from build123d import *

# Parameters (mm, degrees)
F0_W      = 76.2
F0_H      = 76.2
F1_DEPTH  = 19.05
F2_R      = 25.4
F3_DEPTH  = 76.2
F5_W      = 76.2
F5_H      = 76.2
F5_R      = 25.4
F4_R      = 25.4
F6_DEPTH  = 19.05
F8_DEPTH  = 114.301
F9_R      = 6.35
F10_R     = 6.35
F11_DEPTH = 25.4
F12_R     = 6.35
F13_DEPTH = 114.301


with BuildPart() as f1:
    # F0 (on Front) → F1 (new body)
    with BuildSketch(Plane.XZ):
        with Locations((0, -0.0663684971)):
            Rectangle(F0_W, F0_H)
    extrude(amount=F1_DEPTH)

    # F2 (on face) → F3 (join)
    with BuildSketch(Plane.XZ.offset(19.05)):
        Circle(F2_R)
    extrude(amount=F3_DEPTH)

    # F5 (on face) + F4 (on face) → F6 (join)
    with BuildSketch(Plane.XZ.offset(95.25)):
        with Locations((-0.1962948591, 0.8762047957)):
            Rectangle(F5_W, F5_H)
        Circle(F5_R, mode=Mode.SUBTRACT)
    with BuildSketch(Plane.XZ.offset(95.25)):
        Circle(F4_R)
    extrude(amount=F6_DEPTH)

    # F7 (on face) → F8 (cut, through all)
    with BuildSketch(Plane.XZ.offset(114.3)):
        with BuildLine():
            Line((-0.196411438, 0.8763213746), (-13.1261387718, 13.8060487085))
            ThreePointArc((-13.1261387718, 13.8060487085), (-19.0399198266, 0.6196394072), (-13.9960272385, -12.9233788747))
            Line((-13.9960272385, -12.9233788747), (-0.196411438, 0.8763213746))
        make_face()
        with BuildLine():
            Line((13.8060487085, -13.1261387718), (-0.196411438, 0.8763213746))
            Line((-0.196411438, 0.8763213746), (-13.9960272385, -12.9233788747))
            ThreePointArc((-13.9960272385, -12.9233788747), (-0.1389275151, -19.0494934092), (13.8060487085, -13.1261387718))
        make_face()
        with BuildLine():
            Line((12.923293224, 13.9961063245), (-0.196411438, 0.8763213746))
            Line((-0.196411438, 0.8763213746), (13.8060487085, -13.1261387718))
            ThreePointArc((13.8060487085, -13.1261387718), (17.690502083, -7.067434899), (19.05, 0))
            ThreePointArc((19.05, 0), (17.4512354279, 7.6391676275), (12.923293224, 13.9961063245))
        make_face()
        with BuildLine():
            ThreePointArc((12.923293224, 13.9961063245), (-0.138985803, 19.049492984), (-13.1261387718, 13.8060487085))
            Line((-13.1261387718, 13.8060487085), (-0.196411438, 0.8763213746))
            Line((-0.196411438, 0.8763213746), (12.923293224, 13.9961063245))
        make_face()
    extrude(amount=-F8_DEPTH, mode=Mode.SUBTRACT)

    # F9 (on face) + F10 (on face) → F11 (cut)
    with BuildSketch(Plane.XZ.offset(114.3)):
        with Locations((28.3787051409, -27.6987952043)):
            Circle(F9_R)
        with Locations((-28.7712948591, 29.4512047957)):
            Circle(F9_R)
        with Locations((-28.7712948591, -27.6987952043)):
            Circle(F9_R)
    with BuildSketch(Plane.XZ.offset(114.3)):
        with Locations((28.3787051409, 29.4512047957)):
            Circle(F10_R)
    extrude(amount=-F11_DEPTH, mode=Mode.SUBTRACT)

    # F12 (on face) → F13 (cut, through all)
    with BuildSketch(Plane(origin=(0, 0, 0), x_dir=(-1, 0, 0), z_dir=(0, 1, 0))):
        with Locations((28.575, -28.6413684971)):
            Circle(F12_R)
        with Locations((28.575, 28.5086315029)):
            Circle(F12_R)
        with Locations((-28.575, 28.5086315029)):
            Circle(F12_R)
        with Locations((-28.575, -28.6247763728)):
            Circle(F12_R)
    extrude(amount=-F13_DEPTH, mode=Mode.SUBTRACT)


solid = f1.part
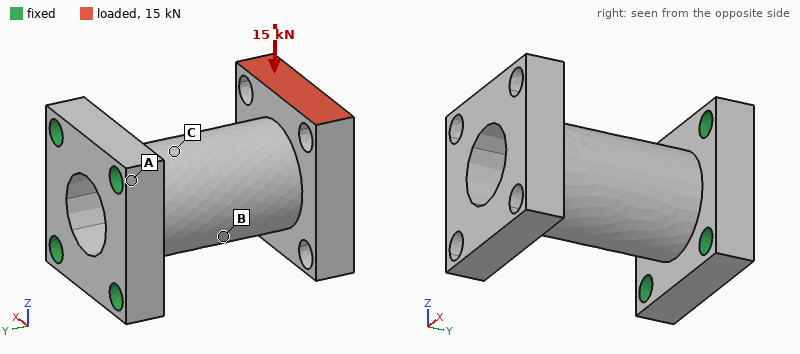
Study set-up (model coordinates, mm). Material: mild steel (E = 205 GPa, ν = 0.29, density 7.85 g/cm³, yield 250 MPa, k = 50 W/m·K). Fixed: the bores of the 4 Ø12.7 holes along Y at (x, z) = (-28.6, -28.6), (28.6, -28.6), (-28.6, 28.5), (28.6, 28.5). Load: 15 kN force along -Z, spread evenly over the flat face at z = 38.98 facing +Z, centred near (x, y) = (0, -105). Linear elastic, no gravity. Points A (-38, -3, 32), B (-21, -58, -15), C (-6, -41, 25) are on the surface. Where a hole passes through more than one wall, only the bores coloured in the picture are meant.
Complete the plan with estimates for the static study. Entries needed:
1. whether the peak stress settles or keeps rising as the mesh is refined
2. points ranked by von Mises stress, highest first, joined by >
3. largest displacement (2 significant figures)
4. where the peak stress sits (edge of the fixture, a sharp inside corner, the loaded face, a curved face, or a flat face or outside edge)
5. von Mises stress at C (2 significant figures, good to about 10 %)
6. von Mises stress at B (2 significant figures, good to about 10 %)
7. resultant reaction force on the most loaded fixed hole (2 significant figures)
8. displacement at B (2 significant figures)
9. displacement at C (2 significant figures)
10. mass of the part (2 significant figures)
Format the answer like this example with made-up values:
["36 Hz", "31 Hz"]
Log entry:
["keeps rising", "C > B > A", "0.18 mm", "edge of the fixture", "99 MPa", "65 MPa", "15 kN", "0.058 mm", "0.040 mm", "1.8 kg"]
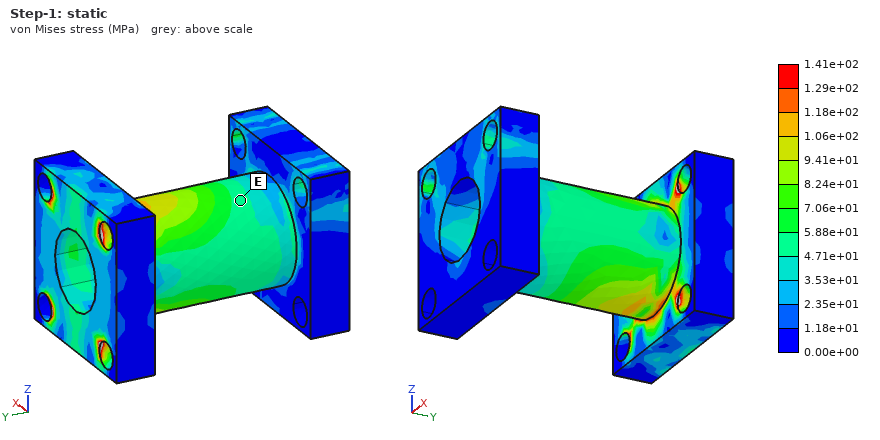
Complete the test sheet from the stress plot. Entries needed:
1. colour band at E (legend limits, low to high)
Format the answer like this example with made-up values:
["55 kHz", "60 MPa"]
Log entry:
["4.71e+01 to 5.88e+01 MPa"]
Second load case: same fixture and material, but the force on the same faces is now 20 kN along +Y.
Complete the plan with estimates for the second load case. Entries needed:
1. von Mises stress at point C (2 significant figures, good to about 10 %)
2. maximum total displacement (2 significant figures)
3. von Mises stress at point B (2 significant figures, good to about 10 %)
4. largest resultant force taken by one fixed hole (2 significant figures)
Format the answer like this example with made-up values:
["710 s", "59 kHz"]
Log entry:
["100 MPa", "0.18 mm", "29 MPa", "14 kN"]
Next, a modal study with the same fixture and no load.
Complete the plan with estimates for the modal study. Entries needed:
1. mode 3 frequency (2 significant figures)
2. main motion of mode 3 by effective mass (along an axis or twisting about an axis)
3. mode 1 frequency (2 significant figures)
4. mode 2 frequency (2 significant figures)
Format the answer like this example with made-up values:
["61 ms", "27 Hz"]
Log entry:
["3700 Hz", "twisting about Y", "1800 Hz", "1800 Hz"]
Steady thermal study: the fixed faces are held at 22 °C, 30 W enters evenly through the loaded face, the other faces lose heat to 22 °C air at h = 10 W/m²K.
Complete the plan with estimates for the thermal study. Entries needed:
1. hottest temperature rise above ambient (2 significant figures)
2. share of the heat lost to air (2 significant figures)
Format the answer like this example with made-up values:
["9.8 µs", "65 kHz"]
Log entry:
["61 K", "39 %"]
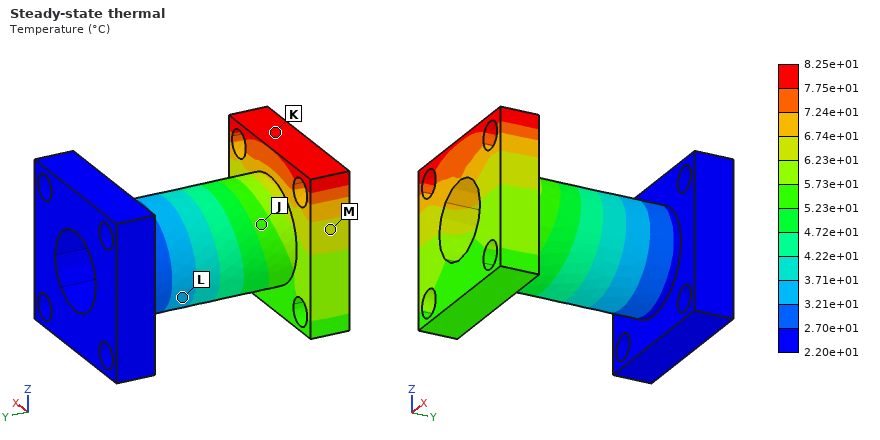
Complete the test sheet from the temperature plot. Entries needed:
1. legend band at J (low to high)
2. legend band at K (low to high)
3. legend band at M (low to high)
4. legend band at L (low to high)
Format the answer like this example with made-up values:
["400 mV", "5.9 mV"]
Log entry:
["5.23e+01 to 5.73e+01 °C", "7.75e+01 to 8.25e+01 °C", "6.23e+01 to 6.74e+01 °C", "3.21e+01 to 3.71e+01 °C"]
